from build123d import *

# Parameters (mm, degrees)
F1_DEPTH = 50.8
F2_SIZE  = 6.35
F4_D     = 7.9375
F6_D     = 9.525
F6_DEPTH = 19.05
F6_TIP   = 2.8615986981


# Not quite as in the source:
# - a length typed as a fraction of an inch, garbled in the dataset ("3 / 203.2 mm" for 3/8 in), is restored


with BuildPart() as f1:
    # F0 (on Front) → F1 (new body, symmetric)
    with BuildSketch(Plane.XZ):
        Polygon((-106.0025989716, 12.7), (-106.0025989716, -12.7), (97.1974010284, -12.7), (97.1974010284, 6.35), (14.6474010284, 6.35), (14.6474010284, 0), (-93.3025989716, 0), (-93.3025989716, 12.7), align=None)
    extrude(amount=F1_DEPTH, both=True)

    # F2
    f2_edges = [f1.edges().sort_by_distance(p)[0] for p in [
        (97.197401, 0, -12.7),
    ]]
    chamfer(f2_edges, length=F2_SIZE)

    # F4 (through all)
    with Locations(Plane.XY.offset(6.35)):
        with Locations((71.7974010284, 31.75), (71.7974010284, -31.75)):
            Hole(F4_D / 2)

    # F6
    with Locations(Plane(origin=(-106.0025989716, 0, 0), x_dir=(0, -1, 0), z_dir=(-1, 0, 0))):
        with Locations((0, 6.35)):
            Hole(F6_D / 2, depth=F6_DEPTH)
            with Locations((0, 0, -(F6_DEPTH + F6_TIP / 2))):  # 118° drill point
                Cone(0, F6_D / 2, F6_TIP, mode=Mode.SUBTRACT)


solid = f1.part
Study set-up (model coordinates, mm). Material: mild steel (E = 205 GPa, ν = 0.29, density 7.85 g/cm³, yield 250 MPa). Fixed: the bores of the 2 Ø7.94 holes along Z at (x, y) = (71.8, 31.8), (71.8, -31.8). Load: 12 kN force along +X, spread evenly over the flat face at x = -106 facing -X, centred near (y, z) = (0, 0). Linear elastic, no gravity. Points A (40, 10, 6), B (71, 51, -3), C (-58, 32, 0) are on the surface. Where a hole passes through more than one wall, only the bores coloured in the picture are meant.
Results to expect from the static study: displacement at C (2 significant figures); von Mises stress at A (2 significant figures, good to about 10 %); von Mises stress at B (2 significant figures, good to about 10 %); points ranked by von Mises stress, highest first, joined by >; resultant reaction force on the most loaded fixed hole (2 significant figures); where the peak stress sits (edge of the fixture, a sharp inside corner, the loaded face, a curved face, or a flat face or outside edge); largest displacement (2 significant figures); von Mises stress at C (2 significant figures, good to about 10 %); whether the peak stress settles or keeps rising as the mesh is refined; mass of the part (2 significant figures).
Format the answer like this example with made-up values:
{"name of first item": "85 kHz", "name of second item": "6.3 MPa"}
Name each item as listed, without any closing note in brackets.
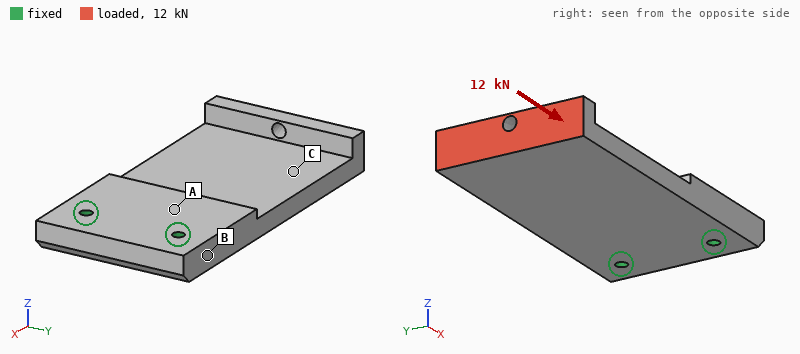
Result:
{"displacement at C": "0.079 mm", "von Mises stress at A": "11 MPa", "von Mises stress at B": "5.4 MPa", "points ranked by von Mises stress, highest first, joined by >": "C > A > B", "resultant reaction force on the most loaded fixed hole": "6.0 kN", "where the peak stress sits": "edge of the fixture", "largest displacement": "0.19 mm", "von Mises stress at C": "36 MPa", "whether the peak stress settles or keeps rising as the mesh is refined": "keeps rising", "mass of the part": "2.6 kg"}
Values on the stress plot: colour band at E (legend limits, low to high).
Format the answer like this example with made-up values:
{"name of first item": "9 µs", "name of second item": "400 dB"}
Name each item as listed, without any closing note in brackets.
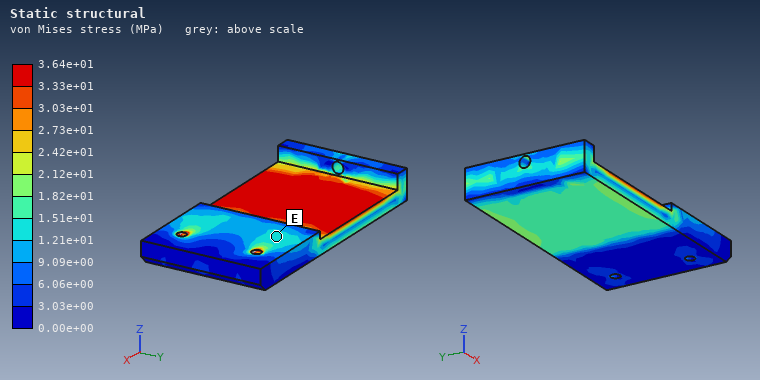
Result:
{"colour band at E": "1.21e+01 to 1.51e+01 MPa"}
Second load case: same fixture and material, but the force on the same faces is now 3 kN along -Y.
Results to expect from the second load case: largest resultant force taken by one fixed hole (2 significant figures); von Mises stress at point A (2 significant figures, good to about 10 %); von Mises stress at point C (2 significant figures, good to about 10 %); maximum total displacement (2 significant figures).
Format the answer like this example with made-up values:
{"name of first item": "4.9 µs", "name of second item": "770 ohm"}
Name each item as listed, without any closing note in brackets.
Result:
{"largest resultant force taken by one fixed hole": "8.1 kN", "von Mises stress at point A": "9.3 MPa", "von Mises stress at point C": "10 MPa", "maximum total displacement": "45 µm"}
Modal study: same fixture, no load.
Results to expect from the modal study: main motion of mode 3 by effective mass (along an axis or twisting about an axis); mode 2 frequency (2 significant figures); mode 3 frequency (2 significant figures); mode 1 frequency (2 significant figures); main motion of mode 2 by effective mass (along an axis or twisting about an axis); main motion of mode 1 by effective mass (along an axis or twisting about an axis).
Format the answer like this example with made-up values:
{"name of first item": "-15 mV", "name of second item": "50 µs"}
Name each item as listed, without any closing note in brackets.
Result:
{"main motion of mode 3 by effective mass": "along Y", "mode 2 frequency": "1400 Hz", "mode 3 frequency": "2100 Hz", "mode 1 frequency": "420 Hz", "main motion of mode 2 by effective mass": "twisting about X", "main motion of mode 1 by effective mass": "along Z"}
